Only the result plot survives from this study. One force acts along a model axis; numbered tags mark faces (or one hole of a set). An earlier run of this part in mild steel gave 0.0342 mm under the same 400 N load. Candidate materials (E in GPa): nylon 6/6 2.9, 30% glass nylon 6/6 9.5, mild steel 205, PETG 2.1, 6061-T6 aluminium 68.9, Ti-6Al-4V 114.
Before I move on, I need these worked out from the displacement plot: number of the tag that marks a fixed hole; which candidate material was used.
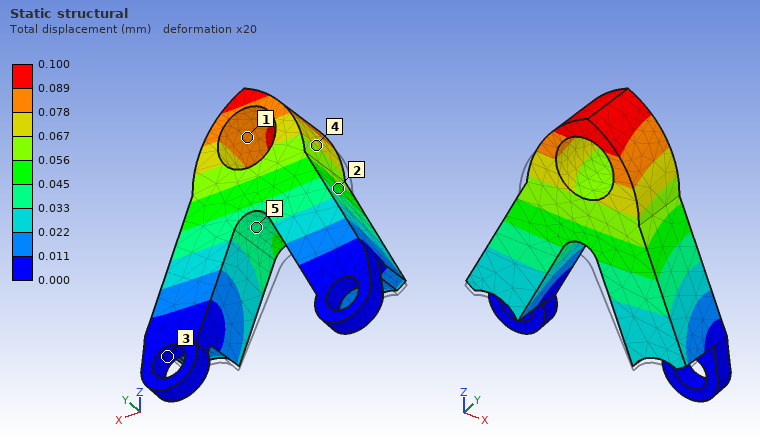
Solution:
3
6061-T6 aluminium
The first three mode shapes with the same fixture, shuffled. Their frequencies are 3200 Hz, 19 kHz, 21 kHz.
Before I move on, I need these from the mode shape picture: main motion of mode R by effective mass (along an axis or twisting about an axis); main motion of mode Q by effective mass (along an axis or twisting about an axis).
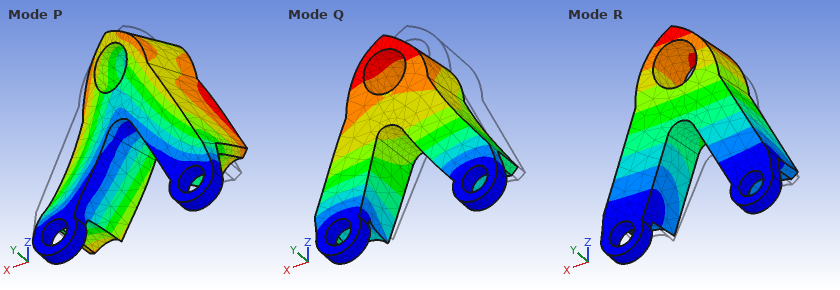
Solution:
along Y
along X
